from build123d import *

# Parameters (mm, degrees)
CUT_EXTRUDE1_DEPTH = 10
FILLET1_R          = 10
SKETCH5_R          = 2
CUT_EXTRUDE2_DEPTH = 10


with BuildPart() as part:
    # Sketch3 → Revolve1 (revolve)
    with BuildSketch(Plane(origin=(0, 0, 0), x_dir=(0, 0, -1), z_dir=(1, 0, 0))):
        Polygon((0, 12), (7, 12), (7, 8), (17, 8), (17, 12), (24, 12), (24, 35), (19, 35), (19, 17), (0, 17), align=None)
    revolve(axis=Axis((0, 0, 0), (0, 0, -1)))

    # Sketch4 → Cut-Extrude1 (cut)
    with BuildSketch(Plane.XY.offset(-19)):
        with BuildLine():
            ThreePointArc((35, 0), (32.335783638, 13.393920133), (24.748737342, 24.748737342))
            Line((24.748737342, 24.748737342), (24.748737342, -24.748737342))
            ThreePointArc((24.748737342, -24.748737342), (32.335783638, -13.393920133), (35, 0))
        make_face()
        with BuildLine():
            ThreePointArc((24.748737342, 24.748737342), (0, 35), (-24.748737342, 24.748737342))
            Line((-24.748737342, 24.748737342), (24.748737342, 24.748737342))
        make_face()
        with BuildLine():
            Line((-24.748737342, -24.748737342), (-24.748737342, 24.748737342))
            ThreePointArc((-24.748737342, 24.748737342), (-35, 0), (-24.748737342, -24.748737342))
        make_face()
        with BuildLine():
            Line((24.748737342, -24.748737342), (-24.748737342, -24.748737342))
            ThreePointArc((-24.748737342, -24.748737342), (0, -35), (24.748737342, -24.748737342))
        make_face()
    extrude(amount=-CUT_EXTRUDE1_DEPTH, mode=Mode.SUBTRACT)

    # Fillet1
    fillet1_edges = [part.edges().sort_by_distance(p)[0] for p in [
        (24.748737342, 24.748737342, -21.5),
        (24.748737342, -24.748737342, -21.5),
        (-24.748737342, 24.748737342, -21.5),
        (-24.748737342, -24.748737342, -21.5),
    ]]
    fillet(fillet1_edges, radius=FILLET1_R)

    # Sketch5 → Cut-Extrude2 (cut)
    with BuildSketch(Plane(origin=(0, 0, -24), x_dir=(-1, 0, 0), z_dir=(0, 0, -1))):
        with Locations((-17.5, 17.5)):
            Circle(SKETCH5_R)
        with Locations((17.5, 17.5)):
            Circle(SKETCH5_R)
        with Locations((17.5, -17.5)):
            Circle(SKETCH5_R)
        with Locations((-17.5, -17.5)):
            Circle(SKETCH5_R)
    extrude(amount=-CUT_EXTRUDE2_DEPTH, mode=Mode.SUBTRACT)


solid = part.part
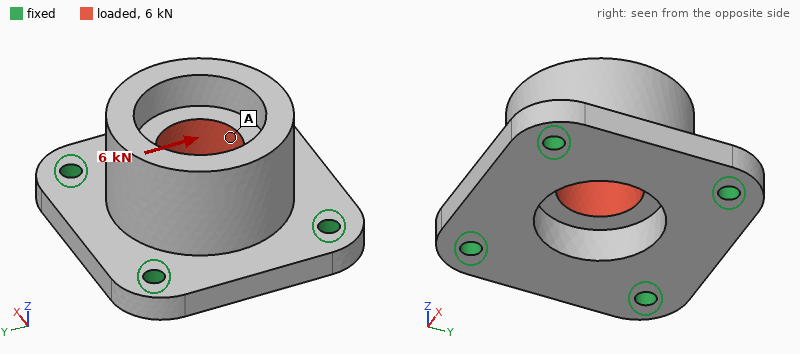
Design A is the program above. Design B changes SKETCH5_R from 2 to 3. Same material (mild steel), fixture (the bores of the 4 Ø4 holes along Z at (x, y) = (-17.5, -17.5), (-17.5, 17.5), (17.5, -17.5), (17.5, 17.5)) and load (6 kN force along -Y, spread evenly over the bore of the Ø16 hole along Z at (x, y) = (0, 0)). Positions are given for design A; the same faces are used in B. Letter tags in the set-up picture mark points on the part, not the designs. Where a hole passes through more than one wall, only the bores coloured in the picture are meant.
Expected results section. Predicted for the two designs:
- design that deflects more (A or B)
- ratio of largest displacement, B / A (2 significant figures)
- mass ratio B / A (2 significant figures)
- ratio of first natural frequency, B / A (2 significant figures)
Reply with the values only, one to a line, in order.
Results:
A
0.82
0.98
1.1
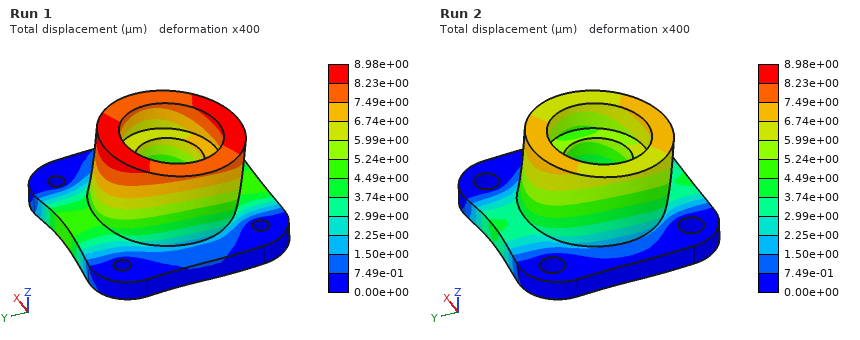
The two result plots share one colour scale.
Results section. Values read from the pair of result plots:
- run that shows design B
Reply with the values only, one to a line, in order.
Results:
Run 2
